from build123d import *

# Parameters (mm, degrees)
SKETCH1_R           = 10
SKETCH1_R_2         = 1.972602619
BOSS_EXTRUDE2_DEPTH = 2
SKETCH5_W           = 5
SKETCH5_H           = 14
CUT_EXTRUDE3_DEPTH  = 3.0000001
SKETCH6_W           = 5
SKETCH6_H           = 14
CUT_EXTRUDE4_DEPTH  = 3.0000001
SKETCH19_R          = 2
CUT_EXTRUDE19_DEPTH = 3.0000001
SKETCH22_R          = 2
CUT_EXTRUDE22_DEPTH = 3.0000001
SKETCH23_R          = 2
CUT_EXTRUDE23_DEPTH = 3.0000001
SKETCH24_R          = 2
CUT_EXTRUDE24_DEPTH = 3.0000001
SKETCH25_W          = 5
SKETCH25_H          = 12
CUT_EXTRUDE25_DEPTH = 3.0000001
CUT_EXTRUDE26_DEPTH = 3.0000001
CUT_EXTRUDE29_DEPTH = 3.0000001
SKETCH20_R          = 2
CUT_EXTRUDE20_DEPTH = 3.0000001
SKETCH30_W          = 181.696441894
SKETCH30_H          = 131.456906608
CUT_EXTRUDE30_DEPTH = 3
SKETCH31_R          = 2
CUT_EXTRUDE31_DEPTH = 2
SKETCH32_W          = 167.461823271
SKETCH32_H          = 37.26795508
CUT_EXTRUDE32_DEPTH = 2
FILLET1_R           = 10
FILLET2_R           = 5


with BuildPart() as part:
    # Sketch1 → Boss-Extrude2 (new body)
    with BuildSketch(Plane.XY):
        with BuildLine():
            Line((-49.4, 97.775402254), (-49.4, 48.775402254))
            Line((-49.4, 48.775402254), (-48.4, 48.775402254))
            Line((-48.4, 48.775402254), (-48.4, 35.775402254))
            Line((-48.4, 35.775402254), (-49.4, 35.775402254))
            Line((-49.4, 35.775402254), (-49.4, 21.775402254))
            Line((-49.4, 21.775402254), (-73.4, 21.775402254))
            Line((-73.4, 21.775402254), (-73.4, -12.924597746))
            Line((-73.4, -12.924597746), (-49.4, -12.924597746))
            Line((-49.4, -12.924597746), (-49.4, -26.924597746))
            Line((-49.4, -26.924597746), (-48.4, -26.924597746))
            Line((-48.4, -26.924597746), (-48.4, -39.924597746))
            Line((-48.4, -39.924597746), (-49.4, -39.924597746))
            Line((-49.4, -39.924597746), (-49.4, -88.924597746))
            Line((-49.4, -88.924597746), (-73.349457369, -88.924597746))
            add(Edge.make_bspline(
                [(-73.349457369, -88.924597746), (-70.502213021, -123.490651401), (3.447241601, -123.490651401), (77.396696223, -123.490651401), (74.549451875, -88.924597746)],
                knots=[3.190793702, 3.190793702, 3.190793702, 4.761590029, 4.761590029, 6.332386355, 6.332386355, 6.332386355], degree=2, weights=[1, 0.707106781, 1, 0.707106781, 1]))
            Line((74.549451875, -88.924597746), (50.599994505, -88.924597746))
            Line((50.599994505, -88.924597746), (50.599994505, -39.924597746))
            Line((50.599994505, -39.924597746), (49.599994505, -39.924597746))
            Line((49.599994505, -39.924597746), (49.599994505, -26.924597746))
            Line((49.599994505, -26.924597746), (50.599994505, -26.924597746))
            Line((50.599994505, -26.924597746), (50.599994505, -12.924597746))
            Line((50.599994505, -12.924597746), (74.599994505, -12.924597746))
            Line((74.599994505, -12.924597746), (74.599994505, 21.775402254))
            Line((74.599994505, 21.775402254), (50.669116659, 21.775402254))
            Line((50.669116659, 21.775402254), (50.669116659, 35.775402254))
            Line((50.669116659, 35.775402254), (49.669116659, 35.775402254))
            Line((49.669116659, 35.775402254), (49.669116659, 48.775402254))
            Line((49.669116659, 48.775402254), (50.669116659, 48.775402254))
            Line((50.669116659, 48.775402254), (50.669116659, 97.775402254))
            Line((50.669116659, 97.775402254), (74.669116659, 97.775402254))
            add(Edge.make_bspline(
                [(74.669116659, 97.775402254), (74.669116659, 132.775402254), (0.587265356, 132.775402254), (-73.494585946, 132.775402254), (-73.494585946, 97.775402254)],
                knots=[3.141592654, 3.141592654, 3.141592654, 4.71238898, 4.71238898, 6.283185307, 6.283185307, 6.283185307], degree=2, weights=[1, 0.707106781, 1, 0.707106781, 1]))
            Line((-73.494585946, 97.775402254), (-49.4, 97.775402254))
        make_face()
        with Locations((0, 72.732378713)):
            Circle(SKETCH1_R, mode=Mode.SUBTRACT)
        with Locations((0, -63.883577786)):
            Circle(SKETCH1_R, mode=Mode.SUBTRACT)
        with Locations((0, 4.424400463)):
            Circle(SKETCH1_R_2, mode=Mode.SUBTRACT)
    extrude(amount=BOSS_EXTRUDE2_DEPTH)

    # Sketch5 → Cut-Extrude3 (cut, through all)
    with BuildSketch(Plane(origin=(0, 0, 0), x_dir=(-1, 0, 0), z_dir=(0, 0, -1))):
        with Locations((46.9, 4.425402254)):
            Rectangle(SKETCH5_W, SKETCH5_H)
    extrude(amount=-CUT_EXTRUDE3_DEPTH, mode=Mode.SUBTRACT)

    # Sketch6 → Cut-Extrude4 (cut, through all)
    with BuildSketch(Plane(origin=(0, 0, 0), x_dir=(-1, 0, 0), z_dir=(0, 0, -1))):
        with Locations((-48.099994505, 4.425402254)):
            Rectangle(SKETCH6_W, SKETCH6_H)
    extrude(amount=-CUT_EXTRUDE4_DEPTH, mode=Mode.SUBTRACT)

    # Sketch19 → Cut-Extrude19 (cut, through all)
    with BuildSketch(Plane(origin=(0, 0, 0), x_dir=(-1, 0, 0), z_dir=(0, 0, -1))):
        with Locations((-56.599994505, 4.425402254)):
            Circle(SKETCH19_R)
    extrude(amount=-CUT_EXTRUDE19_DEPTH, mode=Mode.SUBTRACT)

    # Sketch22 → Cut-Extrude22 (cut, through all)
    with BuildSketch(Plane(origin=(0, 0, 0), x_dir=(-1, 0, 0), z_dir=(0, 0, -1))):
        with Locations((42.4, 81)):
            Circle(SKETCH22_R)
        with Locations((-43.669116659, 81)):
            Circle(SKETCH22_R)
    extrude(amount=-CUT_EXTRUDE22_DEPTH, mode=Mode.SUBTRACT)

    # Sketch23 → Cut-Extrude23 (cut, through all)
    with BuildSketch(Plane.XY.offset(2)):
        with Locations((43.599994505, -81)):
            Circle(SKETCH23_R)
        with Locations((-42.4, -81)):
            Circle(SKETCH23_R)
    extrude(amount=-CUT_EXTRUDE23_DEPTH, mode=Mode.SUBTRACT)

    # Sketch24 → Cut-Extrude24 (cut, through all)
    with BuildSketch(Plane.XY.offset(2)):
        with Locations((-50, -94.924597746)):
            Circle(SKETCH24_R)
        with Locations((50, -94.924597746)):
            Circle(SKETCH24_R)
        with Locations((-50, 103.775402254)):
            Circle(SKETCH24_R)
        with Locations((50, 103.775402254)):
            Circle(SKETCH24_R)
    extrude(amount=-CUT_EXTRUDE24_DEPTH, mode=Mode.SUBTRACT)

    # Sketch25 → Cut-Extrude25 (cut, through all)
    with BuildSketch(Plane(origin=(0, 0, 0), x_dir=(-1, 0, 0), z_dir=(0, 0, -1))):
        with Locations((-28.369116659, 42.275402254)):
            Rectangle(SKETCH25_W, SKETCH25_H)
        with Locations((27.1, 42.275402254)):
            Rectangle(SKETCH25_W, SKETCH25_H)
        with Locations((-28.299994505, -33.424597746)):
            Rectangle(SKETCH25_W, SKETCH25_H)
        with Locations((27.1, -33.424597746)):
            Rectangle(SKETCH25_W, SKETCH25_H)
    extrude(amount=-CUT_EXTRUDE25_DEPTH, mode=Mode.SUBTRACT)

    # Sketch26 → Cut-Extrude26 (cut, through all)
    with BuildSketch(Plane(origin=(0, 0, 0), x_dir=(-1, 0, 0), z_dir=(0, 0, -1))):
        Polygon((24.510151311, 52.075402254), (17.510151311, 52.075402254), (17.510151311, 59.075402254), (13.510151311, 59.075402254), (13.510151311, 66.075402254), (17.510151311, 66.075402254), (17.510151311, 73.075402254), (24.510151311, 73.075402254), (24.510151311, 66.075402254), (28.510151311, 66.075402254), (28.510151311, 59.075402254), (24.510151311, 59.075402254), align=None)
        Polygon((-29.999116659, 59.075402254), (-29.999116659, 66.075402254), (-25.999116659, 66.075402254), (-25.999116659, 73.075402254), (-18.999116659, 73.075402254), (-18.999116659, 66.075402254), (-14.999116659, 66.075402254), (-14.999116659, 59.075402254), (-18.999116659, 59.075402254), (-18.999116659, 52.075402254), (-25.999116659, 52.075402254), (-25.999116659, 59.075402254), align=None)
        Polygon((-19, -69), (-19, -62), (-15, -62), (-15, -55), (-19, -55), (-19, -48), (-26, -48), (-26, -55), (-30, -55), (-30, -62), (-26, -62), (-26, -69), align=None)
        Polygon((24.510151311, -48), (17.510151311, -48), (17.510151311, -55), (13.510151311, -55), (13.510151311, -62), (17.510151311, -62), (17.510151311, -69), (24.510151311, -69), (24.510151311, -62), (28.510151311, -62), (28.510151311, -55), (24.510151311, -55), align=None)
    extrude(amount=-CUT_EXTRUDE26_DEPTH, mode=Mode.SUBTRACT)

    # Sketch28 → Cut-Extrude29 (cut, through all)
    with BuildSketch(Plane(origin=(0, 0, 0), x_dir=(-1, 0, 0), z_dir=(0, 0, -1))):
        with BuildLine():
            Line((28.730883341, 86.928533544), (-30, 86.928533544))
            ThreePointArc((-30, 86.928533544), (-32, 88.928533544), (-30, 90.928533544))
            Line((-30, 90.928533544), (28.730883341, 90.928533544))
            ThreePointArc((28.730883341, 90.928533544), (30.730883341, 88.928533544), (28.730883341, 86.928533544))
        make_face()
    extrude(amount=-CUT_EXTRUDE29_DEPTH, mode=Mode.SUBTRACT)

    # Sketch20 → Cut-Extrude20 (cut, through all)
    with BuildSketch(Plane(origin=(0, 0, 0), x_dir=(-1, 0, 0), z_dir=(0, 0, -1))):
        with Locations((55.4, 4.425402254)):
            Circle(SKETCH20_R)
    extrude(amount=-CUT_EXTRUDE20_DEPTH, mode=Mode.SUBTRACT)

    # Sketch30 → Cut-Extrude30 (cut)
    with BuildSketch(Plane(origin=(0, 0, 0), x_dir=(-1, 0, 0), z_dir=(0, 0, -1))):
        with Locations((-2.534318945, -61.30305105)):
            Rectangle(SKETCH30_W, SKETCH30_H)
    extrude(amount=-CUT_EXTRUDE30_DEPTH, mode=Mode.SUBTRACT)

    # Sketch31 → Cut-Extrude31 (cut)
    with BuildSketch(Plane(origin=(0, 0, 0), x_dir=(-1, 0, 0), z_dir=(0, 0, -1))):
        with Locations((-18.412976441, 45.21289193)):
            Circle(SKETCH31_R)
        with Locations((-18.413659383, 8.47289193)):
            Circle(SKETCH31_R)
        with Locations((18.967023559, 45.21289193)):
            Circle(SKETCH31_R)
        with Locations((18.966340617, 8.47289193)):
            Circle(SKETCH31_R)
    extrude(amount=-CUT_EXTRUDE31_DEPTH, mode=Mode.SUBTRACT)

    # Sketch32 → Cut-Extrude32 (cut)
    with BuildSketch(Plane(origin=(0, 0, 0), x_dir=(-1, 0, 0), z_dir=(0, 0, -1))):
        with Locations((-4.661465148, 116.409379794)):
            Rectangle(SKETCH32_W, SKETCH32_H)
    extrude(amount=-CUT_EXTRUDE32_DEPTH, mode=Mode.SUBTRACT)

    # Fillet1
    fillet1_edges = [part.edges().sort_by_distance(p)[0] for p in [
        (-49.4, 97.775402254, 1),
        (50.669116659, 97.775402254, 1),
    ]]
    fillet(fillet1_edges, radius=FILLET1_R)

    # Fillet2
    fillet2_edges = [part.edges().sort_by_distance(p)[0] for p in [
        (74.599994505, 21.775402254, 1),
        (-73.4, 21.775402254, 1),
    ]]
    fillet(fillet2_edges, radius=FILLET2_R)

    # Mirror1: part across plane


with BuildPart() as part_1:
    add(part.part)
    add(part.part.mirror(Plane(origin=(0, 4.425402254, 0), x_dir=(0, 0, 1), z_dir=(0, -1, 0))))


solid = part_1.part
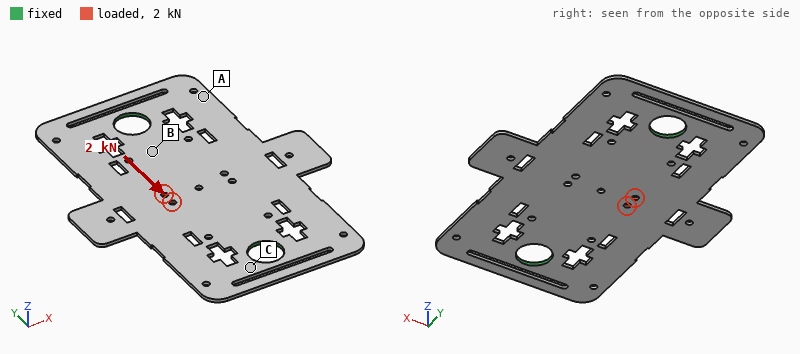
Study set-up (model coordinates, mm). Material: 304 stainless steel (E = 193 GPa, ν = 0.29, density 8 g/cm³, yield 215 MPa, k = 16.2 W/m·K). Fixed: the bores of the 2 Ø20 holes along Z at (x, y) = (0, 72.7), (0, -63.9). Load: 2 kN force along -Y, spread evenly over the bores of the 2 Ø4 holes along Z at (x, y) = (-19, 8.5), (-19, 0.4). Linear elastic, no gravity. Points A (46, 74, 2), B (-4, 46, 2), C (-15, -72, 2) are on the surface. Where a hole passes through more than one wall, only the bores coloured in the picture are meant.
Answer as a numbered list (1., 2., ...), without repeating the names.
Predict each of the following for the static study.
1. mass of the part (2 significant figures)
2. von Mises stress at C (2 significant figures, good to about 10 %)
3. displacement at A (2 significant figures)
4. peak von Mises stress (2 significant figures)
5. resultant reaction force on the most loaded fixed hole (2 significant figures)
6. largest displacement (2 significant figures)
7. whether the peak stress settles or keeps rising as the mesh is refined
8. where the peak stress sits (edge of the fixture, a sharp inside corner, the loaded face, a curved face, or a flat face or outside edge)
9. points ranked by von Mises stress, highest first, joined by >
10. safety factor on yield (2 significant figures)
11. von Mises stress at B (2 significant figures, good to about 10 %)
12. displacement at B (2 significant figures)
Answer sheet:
1. 280 g
2. 7.5 MPa
3. 1.2 µm
4. 90 MPa
5. 1.0 kN
6. 7.0 µm
7. settles
8. the loaded face
9. B > C > A
10. 2.4
11. 15 MPa
12. 1.5 µm
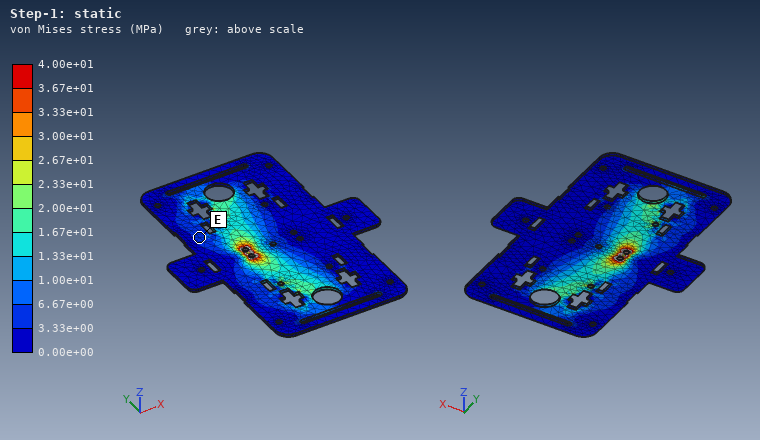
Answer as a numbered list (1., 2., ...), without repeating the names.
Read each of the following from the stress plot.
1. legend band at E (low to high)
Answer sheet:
1. 3.33e+00 to 6.67e+00 MPa
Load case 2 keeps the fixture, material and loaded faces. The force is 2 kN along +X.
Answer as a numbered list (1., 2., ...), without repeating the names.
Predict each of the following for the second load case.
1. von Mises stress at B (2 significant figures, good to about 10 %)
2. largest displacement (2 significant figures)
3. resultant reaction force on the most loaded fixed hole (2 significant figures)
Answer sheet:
1. 17 MPa
2. 12 µm
3. 1.0 kN
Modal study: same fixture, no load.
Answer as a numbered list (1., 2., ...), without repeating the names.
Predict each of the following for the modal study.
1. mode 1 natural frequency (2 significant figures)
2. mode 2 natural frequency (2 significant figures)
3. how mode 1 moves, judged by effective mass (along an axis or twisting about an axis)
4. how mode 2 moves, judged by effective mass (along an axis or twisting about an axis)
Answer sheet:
1. 320 Hz
2. 370 Hz
3. twisting about Y
4. along Z
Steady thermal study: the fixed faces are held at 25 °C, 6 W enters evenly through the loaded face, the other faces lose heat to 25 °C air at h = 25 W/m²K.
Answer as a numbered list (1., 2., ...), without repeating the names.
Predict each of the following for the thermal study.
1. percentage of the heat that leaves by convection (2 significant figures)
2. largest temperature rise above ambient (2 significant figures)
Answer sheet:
1. 92 %
2. 71 K
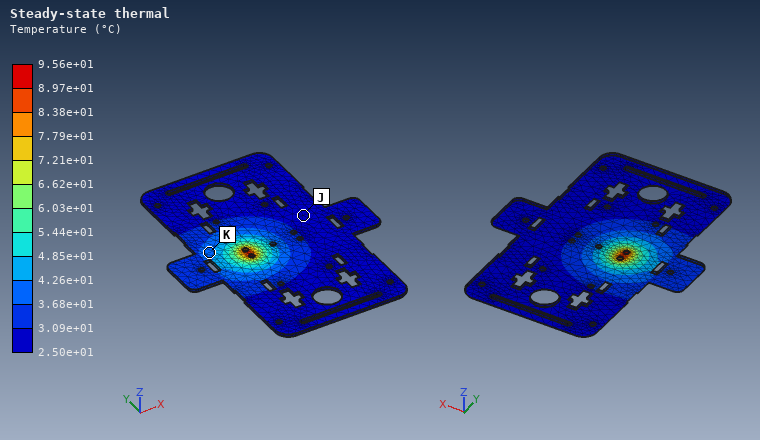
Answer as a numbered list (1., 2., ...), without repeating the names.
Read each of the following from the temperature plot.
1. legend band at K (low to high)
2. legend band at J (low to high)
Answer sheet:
1. 3.68e+01 to 4.26e+01 °C
2. 2.50e+01 to 3.09e+01 °C
